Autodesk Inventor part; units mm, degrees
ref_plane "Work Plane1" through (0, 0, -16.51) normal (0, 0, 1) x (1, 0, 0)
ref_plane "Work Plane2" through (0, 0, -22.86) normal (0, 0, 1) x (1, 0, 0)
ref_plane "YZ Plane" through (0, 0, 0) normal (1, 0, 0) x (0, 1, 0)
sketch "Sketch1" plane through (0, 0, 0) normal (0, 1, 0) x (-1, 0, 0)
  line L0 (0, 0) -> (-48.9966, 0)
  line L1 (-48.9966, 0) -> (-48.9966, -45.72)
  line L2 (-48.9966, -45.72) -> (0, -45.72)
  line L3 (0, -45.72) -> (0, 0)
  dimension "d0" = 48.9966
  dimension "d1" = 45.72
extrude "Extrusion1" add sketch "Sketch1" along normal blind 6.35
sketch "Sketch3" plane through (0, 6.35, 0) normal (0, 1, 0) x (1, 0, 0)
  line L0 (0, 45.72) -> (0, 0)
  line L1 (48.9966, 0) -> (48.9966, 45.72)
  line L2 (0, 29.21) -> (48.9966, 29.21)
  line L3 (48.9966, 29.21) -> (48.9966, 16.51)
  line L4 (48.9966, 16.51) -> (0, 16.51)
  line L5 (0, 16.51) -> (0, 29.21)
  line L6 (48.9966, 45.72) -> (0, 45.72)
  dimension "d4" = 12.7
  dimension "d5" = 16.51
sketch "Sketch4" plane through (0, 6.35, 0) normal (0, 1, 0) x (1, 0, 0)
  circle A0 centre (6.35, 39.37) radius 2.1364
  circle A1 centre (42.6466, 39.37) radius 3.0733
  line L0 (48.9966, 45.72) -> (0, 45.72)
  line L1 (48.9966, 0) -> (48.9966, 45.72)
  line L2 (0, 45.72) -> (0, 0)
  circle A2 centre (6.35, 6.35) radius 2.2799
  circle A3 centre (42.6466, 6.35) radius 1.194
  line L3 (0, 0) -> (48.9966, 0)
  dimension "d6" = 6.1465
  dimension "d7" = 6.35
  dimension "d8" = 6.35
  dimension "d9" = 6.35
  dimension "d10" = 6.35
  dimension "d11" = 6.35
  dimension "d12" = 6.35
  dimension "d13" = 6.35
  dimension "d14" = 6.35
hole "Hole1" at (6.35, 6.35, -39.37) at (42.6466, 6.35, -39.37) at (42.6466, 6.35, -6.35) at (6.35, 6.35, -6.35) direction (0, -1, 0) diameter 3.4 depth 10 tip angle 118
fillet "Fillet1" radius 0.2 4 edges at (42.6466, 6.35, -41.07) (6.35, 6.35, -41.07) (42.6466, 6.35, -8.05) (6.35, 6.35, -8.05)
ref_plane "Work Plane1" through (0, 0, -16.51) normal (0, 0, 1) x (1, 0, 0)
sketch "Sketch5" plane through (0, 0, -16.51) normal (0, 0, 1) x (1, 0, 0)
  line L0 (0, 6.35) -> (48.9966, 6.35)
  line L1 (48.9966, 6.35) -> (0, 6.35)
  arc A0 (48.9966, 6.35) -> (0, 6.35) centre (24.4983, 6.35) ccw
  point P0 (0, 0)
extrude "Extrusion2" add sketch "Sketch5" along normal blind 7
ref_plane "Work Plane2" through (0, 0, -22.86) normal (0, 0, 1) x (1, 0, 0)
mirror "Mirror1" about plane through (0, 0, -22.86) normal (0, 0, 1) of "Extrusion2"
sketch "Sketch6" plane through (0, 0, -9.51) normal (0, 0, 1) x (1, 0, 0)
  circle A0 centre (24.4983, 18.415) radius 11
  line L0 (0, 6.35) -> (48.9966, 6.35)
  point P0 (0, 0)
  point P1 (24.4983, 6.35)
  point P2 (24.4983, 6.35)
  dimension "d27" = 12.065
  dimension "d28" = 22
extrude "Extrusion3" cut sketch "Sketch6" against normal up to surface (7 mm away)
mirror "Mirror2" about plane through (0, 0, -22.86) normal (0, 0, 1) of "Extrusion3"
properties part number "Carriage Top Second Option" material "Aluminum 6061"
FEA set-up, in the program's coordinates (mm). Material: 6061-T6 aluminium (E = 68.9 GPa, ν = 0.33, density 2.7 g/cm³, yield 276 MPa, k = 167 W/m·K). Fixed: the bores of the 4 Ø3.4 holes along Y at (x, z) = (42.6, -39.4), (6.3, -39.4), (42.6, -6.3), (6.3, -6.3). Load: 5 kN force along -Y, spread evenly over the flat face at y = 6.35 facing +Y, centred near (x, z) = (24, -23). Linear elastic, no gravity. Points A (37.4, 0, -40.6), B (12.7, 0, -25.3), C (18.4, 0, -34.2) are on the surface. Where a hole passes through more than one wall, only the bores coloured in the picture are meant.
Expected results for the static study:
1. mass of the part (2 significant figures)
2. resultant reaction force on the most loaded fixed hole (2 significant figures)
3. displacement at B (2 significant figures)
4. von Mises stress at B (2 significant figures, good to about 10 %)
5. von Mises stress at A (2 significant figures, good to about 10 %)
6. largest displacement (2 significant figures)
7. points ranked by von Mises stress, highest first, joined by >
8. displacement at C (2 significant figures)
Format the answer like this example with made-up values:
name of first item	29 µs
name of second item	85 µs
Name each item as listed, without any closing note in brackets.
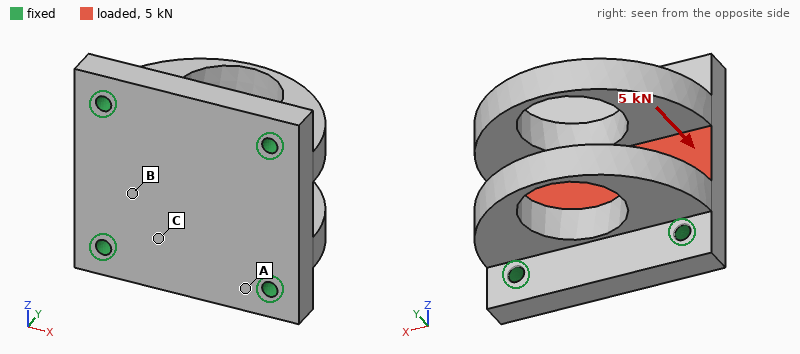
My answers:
mass of the part	59 g
resultant reaction force on the most loaded fixed hole	1.3 kN
displacement at B	22 µm
von Mises stress at B	41 MPa
von Mises stress at A	22 MPa
largest displacement	44 µm
points ranked by von Mises stress, highest first, joined by >	B > A > C
displacement at C	14 µm
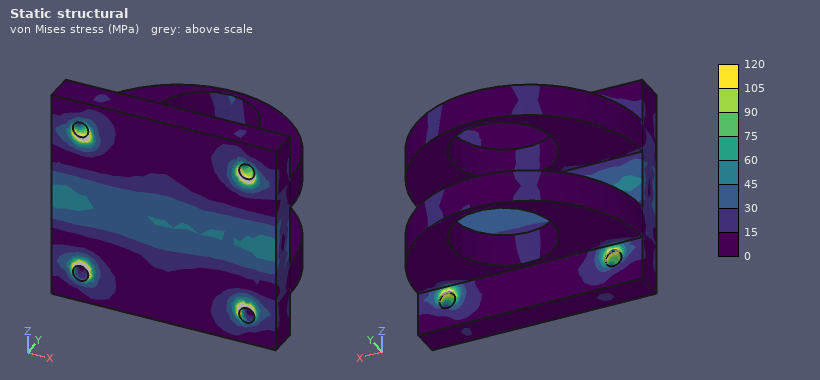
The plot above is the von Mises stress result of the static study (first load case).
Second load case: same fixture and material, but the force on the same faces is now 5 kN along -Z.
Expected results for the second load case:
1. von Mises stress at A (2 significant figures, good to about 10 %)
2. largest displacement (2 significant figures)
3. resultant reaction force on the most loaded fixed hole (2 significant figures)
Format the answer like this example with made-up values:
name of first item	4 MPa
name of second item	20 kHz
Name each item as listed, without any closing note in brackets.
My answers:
von Mises stress at A	8.1 MPa
largest displacement	5.0 µm
resultant reaction force on the most loaded fixed hole	1.3 kN
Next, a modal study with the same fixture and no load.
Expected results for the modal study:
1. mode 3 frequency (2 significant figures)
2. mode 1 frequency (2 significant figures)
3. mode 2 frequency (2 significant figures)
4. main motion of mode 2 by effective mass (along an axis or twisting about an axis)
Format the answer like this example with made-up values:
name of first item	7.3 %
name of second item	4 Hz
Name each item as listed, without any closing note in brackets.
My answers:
mode 3 frequency	13 kHz
mode 1 frequency	8300 Hz
mode 2 frequency	10 kHz
main motion of mode 2 by effective mass	along Z
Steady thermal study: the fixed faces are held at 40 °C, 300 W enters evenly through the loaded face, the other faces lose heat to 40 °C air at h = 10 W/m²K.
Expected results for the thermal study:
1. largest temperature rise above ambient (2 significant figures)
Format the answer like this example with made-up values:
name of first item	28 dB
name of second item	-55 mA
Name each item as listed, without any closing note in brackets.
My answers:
largest temperature rise above ambient	57 K
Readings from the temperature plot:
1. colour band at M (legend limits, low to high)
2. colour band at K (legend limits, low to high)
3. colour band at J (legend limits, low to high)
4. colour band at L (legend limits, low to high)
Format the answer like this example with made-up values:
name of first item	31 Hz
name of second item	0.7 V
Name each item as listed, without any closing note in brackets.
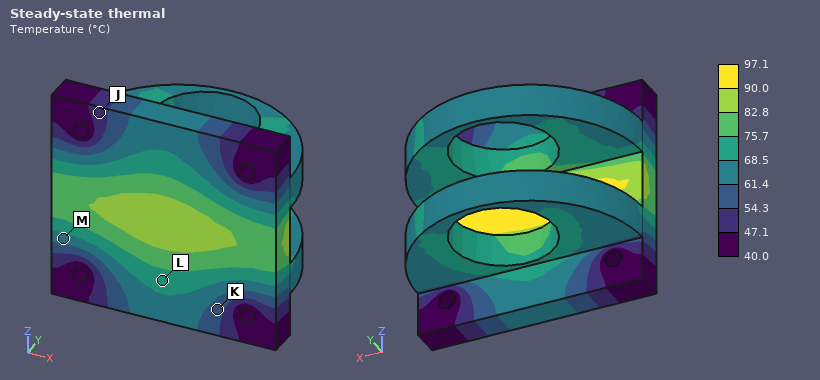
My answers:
colour band at M	61.4 to 68.5 °C
colour band at K	54.3 to 61.4 °C
colour band at J	47.1 to 54.3 °C
colour band at L	68.5 to 75.7 °C
